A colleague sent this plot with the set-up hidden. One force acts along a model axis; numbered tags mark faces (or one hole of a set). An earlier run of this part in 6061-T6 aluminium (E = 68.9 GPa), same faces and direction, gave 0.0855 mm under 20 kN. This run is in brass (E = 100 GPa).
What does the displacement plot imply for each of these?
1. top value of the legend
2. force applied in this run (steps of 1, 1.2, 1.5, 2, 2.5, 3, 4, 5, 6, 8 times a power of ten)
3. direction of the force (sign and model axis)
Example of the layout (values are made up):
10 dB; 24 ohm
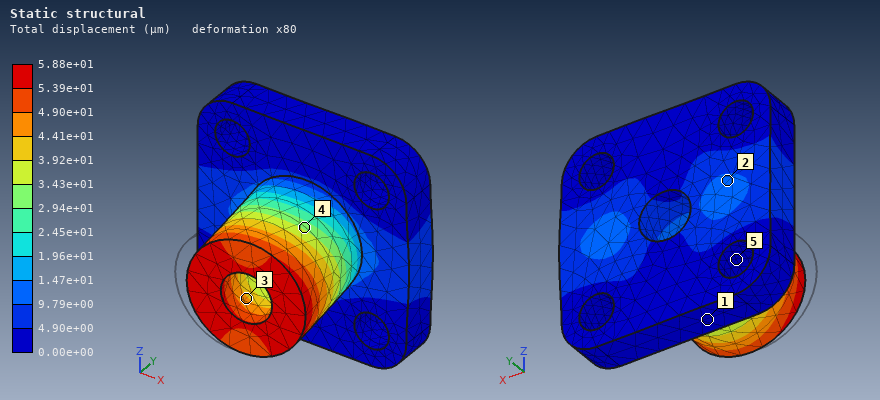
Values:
5.88e+01 µm; 20 kN; +X
